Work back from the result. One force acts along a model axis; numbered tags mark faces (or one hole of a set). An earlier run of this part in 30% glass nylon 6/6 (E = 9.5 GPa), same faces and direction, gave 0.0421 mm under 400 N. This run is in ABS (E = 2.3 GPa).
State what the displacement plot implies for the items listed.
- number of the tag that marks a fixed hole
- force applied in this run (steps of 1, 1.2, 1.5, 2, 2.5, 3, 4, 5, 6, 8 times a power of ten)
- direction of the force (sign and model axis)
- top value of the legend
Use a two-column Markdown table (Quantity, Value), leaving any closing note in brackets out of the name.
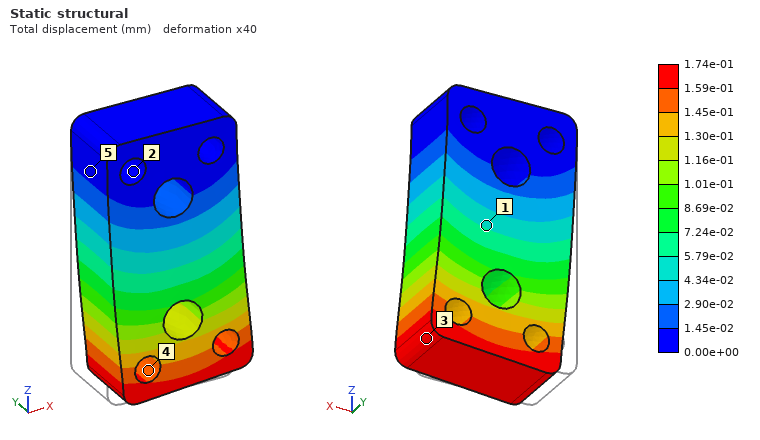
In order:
| Quantity | Value |
|---|---|
| number of the tag that marks a fixed hole | 2 |
| force applied in this run | 400 N |
| direction of the force | +X |
| top value of the legend | 1.74e-01 mm |
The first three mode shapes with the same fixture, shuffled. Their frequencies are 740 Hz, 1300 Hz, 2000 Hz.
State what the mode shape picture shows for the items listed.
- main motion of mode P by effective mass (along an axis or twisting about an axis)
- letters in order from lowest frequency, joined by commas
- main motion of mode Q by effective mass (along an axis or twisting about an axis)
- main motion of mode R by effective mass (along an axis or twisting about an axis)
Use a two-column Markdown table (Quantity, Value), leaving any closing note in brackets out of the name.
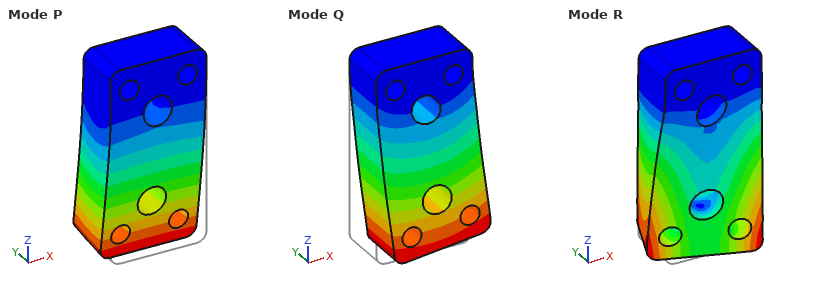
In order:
| Quantity | Value |
|---|---|
| main motion of mode P by effective mass | along Y |
| letters in order from lowest frequency, joined by commas | P, Q, R |
| main motion of mode Q by effective mass | along X |
| main motion of mode R by effective mass | twisting about Z |
